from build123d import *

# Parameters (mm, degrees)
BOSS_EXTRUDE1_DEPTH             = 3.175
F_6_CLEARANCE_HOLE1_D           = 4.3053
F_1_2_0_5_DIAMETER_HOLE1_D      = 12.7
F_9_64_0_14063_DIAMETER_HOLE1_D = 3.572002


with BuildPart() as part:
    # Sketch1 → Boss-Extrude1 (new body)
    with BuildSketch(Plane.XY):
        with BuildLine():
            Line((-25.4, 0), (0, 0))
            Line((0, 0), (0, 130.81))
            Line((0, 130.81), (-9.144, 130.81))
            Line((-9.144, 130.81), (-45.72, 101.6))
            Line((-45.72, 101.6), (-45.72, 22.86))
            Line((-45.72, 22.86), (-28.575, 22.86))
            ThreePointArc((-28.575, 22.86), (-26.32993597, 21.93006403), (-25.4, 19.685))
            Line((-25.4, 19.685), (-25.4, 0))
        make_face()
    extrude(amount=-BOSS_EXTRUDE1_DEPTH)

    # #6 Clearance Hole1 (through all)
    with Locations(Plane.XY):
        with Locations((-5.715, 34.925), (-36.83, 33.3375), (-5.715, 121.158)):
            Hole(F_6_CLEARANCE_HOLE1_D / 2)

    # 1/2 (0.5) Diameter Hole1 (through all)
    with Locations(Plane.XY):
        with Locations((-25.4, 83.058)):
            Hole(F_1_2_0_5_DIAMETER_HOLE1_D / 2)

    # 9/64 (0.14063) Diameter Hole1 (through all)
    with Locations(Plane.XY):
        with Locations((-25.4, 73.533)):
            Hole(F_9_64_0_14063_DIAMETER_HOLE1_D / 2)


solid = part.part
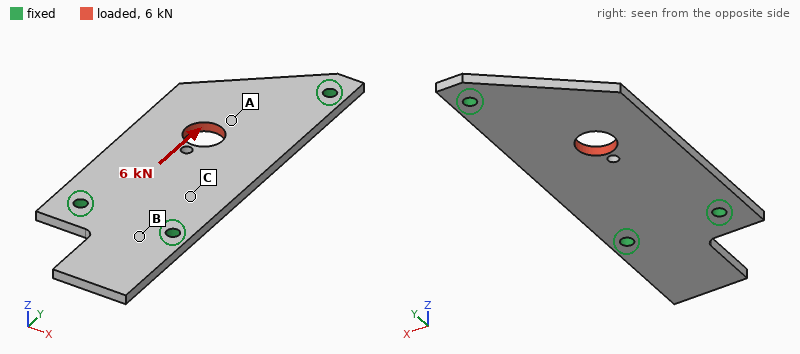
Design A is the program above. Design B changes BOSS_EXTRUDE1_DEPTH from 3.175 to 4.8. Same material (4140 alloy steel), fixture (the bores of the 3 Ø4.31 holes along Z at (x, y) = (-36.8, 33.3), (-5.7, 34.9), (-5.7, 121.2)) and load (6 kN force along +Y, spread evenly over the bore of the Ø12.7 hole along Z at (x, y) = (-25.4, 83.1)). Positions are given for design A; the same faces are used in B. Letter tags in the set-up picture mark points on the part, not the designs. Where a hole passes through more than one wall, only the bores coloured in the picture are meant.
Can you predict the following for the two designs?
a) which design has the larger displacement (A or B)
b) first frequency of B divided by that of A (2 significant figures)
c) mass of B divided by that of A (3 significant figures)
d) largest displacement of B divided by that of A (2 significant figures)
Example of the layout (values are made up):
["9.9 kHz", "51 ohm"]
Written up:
["A", "1.5", "1.51", "0.66"]
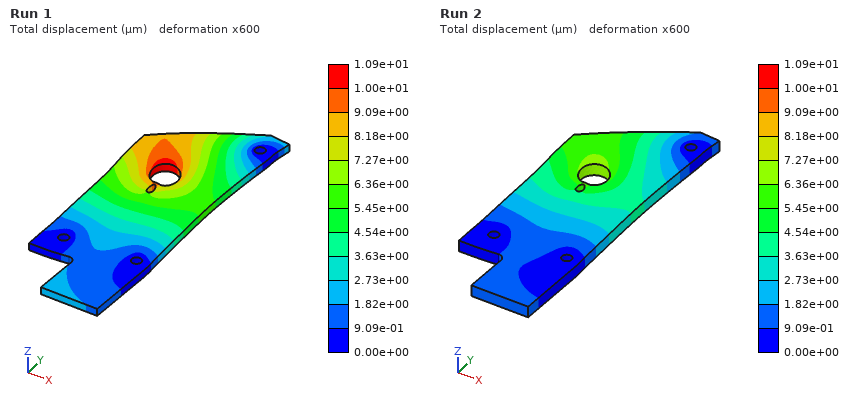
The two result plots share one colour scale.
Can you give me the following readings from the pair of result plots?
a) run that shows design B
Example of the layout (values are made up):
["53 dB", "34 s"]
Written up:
["Run 2"]
